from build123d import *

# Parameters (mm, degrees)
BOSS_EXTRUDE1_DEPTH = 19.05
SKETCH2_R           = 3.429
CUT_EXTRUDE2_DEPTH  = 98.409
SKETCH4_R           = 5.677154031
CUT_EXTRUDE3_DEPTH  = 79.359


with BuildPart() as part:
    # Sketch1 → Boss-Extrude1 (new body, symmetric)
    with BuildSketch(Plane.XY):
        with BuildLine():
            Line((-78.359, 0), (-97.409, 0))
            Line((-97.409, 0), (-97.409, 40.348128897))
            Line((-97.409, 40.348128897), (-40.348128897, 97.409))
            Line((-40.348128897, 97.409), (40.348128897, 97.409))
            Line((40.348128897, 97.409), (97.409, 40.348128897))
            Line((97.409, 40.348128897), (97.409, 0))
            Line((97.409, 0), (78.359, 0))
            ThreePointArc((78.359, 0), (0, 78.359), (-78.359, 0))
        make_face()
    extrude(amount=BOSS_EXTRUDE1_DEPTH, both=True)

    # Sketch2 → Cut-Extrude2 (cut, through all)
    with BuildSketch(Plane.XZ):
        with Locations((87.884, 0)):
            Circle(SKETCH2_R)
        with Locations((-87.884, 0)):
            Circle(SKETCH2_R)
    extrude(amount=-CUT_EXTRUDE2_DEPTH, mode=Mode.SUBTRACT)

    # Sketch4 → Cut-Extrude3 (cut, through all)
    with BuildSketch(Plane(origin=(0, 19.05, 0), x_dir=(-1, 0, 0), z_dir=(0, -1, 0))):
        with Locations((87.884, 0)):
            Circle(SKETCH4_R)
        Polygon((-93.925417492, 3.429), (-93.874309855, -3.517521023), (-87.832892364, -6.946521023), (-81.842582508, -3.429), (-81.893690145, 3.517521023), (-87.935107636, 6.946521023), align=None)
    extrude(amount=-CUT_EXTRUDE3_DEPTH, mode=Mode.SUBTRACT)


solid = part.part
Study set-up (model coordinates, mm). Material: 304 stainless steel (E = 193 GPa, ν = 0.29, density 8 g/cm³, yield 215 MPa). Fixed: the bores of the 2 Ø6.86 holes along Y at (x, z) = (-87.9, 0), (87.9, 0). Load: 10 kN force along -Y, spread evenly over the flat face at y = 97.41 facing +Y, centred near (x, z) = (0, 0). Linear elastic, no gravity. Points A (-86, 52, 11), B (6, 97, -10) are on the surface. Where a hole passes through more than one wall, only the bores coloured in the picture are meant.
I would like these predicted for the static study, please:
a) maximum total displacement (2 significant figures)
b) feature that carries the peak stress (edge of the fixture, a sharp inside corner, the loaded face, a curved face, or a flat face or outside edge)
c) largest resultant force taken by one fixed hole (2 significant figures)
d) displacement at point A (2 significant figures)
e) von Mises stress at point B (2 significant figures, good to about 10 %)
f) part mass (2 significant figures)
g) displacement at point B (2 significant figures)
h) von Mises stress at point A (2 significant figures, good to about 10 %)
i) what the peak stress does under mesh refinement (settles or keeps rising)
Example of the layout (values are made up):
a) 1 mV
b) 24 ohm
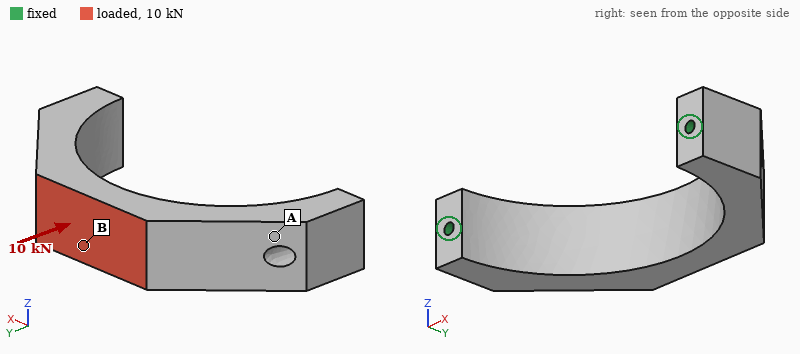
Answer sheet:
a) 20 µm
b) edge of the fixture
c) 6.4 kN
d) 6.1 µm
e) 29 MPa
f) 1.8 kg
g) 19 µm
h) 7.1 MPa
i) keeps rising
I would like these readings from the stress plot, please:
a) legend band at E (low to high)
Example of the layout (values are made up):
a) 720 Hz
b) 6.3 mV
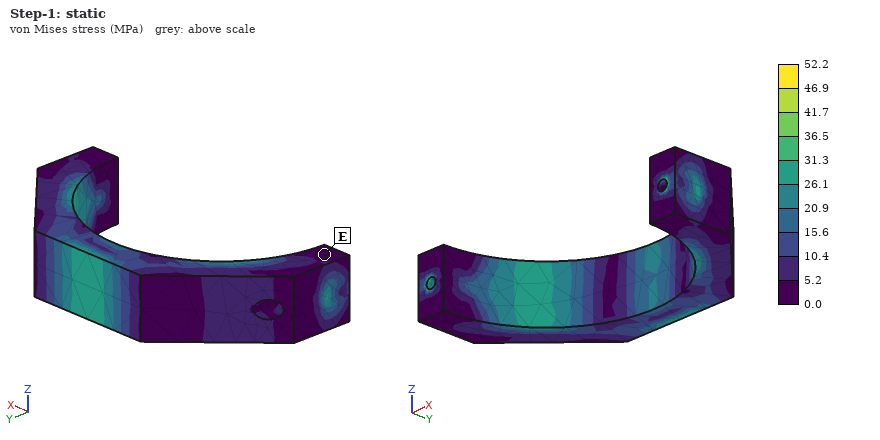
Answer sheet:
a) 0.0 to 5.2 MPa
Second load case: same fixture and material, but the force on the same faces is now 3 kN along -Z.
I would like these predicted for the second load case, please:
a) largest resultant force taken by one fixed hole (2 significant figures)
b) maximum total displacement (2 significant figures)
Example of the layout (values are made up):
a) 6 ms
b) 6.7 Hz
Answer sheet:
a) 1.5 kN
b) 67 µm
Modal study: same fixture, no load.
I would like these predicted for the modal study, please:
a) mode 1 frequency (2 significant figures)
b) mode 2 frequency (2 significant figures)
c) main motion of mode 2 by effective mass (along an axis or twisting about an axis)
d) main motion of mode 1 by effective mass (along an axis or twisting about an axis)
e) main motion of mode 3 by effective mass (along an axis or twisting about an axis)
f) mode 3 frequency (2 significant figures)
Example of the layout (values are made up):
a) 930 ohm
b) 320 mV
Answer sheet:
a) 1400 Hz
b) 2500 Hz
c) along X
d) along Z
e) twisting about Y
f) 3700 Hz
